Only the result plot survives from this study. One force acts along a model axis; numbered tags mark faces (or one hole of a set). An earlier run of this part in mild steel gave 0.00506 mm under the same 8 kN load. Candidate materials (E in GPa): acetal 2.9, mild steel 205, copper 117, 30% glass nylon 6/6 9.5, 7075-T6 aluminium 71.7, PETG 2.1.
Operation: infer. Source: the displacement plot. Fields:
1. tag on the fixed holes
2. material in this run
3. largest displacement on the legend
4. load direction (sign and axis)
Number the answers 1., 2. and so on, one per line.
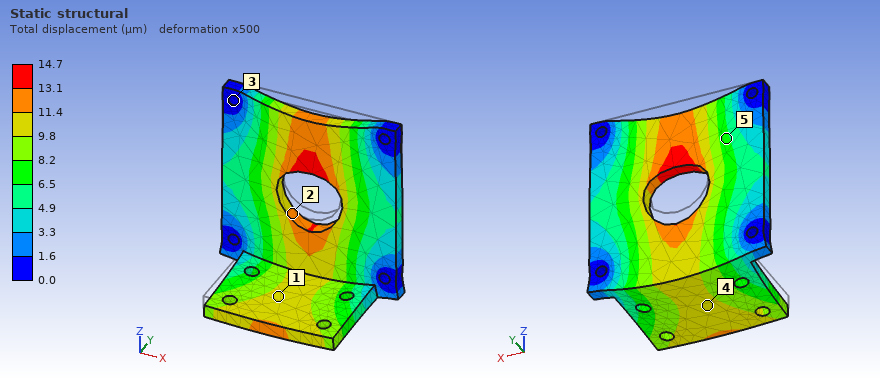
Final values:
1. 3
2. 7075-T6 aluminium
3. 14.7 µm
4. -Z
